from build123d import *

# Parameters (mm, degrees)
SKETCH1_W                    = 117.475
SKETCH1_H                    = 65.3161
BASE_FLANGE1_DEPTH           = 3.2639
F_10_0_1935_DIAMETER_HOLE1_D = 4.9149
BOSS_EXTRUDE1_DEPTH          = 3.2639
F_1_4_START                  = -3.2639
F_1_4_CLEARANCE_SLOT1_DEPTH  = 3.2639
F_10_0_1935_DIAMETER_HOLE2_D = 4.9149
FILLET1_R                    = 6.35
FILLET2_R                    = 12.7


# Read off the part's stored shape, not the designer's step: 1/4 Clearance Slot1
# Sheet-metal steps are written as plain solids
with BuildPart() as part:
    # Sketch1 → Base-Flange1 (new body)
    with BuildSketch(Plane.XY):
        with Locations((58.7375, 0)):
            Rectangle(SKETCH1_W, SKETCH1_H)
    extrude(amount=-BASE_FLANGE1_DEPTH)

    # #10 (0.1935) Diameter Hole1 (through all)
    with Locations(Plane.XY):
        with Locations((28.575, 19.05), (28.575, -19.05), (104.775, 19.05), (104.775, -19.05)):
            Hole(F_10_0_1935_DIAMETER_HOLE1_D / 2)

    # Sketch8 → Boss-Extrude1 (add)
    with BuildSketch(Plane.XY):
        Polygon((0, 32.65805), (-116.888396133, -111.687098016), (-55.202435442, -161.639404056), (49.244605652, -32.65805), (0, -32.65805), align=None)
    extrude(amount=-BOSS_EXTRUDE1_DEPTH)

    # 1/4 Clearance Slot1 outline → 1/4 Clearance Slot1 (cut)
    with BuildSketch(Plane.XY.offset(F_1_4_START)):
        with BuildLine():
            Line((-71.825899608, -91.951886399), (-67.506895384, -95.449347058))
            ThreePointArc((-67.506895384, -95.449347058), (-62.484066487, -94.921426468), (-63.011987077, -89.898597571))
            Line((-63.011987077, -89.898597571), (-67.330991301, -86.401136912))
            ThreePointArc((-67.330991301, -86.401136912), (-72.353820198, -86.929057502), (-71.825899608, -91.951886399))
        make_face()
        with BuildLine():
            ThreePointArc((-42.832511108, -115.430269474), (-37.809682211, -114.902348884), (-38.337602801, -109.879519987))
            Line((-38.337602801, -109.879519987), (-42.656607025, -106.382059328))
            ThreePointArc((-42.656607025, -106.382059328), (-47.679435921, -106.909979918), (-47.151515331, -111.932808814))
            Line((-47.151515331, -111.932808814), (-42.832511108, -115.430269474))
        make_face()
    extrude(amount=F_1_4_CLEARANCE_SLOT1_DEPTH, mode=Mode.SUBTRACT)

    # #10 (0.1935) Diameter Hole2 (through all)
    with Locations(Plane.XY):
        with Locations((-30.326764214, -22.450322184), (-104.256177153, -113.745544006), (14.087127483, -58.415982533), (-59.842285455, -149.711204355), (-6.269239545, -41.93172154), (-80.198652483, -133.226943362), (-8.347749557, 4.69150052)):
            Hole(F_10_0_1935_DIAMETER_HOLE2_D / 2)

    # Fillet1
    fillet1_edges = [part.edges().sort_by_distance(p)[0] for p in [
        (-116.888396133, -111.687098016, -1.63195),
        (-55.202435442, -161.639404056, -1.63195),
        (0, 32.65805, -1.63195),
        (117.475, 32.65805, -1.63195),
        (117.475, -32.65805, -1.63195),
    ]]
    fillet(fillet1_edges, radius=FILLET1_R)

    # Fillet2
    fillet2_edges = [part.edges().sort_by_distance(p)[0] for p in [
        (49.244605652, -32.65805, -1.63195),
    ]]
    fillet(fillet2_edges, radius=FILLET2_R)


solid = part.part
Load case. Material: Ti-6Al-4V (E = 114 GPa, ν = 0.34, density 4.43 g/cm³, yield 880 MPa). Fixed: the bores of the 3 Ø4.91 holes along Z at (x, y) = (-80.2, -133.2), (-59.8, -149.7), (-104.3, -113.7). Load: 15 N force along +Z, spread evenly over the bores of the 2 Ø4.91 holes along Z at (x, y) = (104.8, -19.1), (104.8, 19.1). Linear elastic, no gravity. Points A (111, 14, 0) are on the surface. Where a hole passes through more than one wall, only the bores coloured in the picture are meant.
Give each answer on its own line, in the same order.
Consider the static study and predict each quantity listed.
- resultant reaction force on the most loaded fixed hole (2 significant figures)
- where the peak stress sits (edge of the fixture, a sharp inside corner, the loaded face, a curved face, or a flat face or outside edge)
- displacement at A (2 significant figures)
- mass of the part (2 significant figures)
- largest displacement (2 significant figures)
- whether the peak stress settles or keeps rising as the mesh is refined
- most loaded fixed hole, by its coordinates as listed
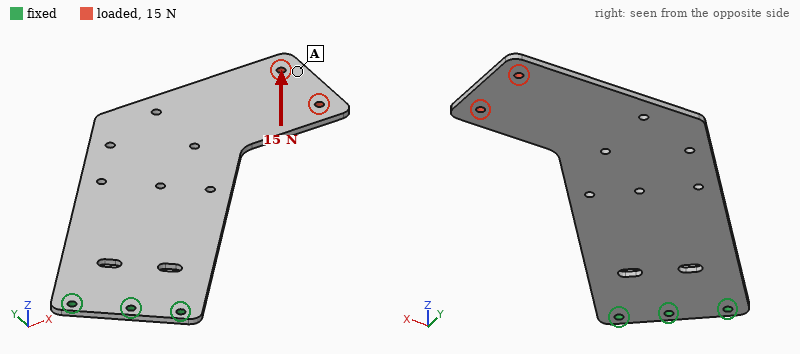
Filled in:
27 N
edge of the fixture
2.6 mm
280 g
2.8 mm
keeps rising
(-80.2, -133.2)
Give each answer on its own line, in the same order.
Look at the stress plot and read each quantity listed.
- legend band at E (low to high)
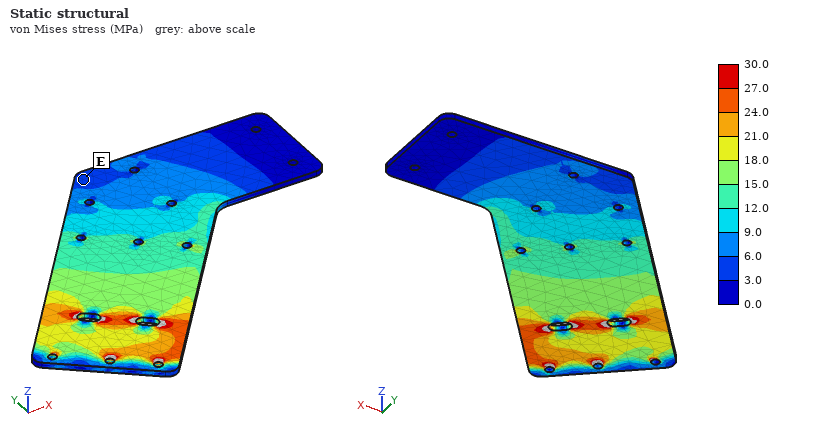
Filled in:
3.0 to 6.0 MPa
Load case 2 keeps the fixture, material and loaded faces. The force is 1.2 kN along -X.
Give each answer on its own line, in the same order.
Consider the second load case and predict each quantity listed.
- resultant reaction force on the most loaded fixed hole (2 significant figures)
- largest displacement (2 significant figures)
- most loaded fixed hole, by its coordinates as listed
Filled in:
3.0 kN
0.22 mm
(-104.3, -113.7)
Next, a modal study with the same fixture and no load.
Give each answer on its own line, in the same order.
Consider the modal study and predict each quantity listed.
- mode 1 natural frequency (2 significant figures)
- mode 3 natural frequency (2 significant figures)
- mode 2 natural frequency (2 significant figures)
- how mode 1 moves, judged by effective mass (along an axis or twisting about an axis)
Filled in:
45 Hz
360 Hz
200 Hz
along Z
